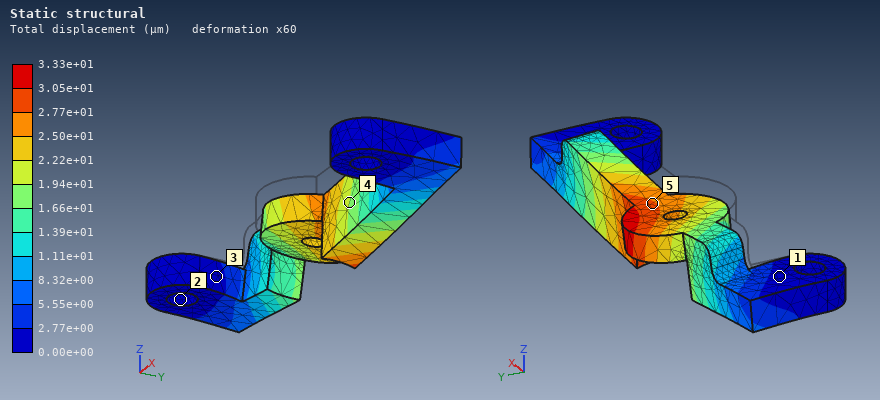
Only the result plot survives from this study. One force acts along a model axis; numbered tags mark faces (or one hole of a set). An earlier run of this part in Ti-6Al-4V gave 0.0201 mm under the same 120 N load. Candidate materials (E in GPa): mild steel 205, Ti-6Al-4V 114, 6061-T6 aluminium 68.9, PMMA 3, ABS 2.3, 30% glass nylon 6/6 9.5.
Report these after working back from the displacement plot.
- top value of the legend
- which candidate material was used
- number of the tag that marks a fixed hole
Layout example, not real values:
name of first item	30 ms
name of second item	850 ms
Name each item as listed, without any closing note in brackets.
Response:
top value of the legend	3.33e+01 µm
which candidate material was used	6061-T6 aluminium
number of the tag that marks a fixed hole	2
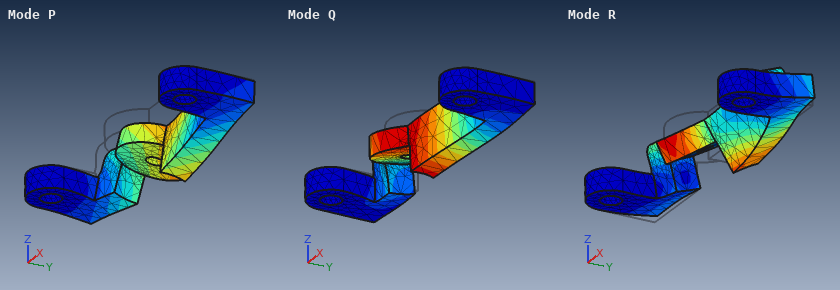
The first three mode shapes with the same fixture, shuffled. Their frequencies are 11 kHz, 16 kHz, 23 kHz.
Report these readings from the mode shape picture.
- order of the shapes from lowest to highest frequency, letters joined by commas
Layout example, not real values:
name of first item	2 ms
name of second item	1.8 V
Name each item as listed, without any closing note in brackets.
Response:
order of the shapes from lowest to highest frequency, letters joined by commas	P, Q, R
